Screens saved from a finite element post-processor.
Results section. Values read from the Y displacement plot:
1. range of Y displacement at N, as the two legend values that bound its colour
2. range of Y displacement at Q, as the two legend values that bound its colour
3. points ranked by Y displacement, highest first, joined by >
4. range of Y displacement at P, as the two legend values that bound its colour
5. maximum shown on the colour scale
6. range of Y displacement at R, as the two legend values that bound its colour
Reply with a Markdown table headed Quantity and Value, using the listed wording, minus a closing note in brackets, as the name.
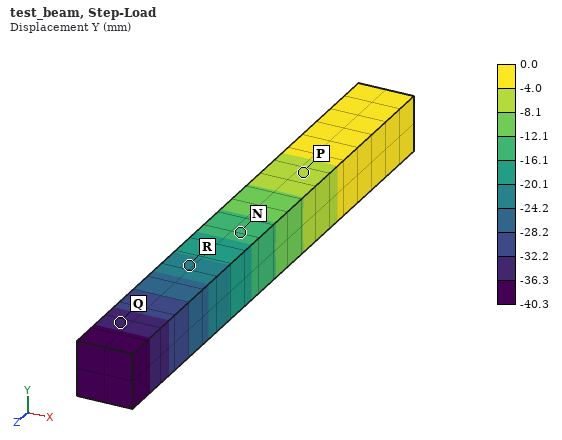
| Quantity | Value |
|---|---|
| range of Y displacement at N, as the two legend values that bound its colour | -16.1 to -12.1 mm |
| range of Y displacement at Q, as the two legend values that bound its colour | -36.3 to -32.2 mm |
| points ranked by Y displacement, highest first, joined by > | P > N > R > Q |
| range of Y displacement at P, as the two legend values that bound its colour | -8.1 to -4.0 mm |
| maximum shown on the colour scale | 0.0 mm |
| range of Y displacement at R, as the two legend values that bound its colour | -24.2 to -20.1 mm |
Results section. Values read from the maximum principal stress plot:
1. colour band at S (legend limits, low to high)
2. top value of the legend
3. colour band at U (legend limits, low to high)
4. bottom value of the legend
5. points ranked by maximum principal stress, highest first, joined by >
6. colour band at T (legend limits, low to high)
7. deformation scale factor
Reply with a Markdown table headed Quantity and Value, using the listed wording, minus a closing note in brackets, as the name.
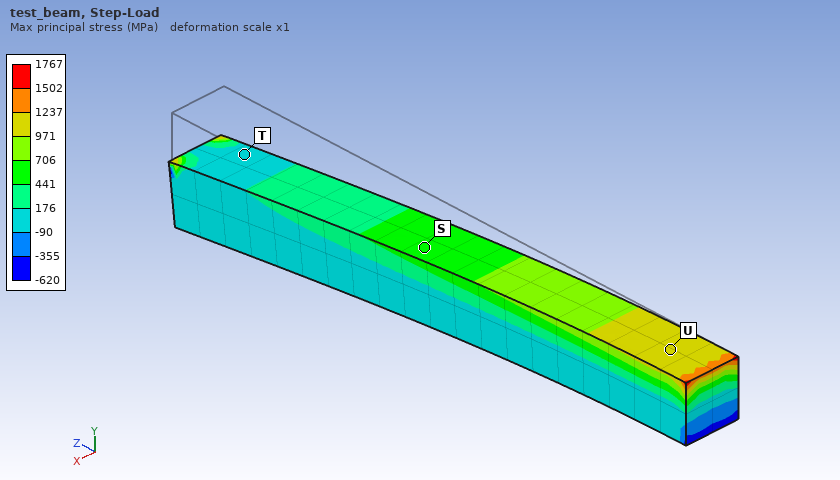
| Quantity | Value |
|---|---|
| colour band at S | 441 to 706 MPa |
| top value of the legend | 1767 MPa |
| colour band at U | 971 to 1237 MPa |
| bottom value of the legend | -620 MPa |
| points ranked by maximum principal stress, highest first, joined by > | U > S > T |
| colour band at T | -90 to 176 MPa |
| deformation scale factor | 1 |
